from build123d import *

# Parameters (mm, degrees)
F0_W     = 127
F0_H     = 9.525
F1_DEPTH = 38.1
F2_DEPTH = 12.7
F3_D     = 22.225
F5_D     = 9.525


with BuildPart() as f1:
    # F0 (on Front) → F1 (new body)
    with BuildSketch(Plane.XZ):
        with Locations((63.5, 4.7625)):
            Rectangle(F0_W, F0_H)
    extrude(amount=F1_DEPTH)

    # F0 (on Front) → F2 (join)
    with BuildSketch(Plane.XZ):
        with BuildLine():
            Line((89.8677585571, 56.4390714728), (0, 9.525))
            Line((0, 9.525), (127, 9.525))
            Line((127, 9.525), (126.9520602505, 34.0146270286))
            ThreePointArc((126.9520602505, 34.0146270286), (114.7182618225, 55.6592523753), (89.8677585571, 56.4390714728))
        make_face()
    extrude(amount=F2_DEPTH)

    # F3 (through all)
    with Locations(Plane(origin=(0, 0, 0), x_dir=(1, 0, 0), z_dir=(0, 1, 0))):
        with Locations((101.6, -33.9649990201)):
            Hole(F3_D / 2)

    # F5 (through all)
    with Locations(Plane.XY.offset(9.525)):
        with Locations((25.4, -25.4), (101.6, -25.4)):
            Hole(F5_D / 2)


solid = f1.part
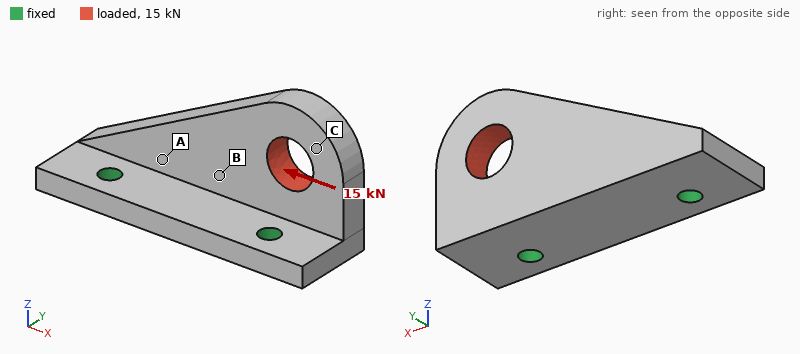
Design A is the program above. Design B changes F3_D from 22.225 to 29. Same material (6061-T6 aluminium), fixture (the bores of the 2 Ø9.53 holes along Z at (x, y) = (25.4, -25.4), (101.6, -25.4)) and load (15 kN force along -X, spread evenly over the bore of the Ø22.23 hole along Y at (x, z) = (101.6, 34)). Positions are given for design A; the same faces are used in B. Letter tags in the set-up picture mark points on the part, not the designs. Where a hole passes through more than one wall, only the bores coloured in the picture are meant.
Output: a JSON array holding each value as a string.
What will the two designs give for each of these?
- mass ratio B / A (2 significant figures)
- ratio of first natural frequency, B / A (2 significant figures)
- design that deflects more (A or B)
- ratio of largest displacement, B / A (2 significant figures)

["0.96", "1.0", "B", "1.1"]
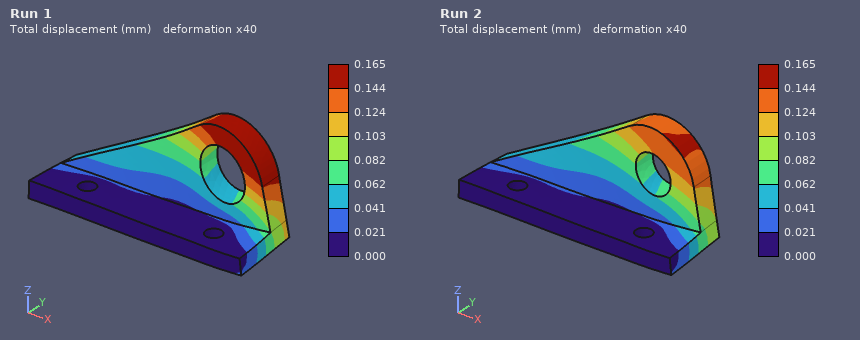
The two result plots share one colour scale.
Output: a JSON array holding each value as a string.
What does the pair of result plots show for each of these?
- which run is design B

["Run 1"]
